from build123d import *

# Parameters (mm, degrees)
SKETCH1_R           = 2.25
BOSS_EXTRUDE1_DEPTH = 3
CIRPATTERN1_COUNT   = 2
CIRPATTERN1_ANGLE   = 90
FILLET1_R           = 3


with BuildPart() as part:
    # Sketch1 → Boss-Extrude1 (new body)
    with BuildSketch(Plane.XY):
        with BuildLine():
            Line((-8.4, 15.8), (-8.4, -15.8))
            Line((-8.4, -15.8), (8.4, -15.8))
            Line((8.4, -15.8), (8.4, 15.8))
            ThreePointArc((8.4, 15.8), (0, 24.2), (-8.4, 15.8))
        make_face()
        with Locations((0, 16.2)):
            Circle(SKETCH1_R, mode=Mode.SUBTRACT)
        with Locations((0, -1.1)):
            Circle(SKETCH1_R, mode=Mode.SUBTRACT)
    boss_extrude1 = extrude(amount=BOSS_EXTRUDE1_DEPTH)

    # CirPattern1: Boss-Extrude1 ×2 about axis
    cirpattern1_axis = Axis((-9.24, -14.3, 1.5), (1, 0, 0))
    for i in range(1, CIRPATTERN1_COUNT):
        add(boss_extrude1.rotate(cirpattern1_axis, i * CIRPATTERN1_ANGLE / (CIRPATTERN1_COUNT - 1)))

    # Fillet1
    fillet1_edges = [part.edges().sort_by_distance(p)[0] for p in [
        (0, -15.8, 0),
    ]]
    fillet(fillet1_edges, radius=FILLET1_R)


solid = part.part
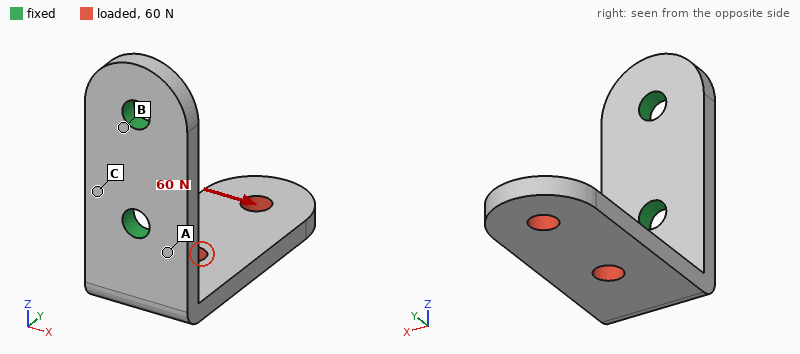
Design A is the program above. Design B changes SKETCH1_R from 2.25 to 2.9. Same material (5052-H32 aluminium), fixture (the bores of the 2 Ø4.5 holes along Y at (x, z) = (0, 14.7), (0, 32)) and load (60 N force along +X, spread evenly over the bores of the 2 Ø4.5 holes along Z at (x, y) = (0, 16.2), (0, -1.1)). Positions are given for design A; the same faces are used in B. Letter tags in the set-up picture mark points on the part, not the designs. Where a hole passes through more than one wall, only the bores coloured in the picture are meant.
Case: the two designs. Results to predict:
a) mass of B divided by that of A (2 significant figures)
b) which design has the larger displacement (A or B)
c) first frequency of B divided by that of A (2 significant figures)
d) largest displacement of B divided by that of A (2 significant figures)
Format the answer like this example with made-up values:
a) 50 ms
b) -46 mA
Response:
a) 0.96
b) A
c) 1.0
d) 0.89
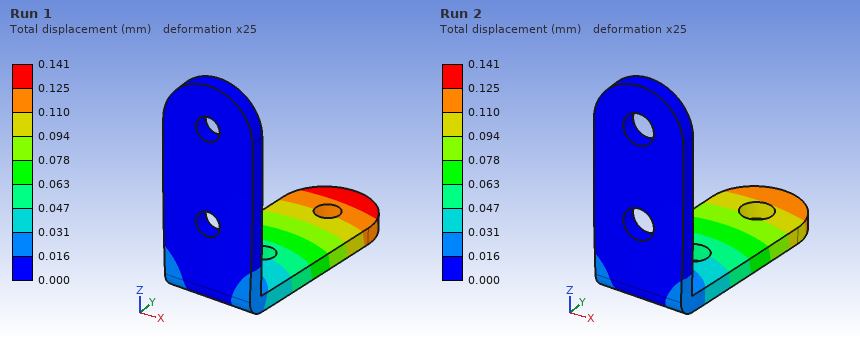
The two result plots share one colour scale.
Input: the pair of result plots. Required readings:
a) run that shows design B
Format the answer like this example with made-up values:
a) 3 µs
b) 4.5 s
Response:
a) Run 2
